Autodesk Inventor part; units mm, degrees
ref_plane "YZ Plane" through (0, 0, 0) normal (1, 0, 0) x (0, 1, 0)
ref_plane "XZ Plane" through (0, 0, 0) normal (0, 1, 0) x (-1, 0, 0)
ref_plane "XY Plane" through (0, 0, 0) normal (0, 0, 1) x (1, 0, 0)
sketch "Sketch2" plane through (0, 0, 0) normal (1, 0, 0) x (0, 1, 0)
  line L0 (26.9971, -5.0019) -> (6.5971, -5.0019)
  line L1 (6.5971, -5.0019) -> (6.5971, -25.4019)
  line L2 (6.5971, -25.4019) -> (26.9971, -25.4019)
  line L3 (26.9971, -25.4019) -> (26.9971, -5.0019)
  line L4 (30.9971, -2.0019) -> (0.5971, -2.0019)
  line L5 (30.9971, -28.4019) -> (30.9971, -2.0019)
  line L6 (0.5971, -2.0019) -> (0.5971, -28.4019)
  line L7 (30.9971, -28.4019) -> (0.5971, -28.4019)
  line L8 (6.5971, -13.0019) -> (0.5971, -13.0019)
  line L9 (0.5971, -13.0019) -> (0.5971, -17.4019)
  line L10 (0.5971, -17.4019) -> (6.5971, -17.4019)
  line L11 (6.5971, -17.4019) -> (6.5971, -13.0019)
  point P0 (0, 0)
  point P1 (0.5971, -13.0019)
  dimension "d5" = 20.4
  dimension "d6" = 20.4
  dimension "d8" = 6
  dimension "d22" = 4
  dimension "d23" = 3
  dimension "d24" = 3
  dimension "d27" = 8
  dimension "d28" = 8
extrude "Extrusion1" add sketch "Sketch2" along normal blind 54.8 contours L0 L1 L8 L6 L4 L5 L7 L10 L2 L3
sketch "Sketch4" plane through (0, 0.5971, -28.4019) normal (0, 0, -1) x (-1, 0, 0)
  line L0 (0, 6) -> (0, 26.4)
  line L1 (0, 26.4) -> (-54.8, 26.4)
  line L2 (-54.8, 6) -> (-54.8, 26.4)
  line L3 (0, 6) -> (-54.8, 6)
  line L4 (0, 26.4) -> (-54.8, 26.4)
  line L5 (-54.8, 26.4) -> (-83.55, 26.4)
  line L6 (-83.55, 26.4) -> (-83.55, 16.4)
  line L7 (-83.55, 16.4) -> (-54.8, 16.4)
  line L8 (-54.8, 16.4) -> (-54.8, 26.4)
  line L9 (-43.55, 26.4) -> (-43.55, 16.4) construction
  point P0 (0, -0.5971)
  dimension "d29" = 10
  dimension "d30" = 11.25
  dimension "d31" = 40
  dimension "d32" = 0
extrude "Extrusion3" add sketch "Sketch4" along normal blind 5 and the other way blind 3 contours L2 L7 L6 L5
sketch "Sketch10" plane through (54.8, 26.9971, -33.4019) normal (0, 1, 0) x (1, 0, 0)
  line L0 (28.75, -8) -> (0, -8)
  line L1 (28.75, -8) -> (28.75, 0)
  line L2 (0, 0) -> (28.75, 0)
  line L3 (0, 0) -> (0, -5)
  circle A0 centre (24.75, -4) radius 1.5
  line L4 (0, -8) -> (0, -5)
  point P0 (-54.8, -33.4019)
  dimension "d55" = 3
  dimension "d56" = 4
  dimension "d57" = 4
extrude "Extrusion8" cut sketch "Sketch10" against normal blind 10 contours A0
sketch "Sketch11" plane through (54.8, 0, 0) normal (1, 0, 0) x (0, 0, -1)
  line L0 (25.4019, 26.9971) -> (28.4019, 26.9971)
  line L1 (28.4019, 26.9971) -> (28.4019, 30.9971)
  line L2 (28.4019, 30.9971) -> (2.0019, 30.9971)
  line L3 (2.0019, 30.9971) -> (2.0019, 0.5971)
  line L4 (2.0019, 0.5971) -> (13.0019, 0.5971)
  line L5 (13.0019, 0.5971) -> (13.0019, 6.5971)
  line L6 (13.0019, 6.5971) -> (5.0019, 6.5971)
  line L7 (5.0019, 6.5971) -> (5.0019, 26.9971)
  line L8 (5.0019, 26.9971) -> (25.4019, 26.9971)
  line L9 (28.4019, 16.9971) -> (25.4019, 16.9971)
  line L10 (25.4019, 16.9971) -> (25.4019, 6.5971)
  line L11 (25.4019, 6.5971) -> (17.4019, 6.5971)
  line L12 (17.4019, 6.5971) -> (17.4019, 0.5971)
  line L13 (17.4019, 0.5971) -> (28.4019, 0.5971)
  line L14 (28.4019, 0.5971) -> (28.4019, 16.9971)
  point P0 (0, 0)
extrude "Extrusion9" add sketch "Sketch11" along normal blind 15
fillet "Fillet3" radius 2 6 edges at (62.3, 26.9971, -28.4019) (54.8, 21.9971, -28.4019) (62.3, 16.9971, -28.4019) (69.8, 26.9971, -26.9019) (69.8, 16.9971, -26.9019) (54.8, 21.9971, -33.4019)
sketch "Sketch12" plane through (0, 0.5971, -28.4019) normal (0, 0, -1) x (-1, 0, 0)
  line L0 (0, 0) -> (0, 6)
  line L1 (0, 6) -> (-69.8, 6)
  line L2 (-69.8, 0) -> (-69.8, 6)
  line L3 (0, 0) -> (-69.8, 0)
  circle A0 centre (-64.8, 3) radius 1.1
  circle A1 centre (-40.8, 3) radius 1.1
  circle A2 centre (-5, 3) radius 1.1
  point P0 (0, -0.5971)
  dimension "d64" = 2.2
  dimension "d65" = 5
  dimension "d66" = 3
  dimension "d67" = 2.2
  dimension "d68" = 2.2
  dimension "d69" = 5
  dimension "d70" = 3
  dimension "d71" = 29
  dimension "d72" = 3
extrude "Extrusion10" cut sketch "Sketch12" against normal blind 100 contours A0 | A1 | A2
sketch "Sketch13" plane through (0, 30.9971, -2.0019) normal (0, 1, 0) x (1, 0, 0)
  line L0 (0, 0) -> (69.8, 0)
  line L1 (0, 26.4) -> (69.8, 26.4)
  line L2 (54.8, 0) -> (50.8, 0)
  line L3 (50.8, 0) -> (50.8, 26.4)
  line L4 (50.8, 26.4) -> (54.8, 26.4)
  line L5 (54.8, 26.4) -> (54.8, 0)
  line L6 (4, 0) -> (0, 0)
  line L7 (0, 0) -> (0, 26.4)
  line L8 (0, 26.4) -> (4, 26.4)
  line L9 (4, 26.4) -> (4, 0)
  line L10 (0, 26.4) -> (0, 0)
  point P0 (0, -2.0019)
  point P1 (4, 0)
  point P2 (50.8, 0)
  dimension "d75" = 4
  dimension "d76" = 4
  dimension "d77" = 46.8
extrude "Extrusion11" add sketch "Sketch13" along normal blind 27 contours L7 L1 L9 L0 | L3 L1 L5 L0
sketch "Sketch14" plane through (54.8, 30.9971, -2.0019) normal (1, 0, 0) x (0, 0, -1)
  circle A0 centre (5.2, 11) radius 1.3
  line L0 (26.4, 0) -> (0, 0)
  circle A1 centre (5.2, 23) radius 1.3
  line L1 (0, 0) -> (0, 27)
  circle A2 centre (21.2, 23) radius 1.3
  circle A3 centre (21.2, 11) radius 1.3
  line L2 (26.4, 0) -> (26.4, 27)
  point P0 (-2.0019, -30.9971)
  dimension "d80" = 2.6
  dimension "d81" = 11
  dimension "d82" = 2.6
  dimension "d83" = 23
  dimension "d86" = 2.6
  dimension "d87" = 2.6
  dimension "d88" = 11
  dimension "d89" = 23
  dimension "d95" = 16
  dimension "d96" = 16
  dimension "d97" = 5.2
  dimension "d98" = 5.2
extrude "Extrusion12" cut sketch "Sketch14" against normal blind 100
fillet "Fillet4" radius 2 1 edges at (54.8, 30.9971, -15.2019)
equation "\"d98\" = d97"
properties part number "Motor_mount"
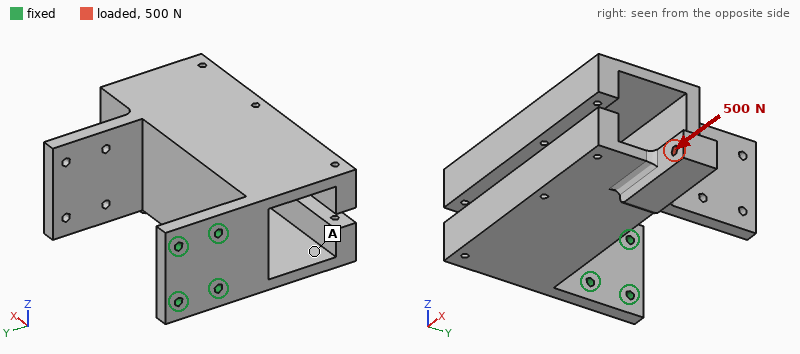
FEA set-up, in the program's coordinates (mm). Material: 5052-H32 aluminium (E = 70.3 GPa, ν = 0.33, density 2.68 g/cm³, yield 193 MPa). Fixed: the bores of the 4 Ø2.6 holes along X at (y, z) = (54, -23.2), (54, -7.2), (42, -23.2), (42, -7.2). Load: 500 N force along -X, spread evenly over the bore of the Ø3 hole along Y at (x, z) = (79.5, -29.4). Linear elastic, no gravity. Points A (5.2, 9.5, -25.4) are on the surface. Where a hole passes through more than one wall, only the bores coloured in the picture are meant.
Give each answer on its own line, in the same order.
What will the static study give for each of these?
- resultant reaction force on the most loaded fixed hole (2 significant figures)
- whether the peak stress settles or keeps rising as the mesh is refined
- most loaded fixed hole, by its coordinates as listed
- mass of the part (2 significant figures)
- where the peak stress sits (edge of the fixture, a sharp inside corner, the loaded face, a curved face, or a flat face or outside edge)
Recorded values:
780 N
keeps rising
(42, -23.2)
86 g
edge of the fixture
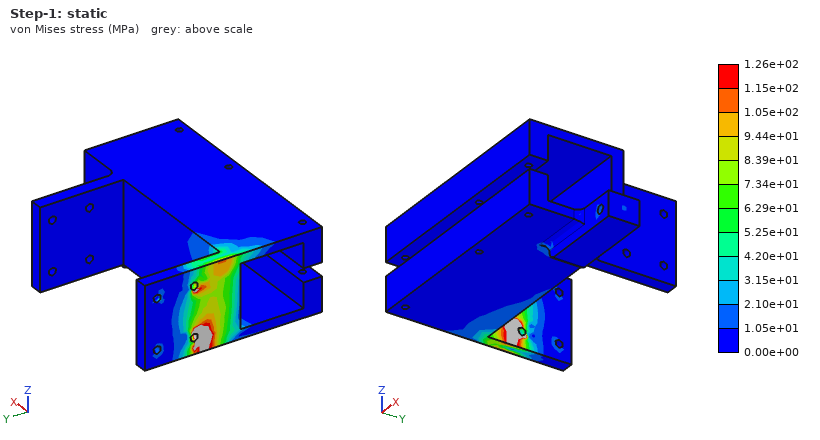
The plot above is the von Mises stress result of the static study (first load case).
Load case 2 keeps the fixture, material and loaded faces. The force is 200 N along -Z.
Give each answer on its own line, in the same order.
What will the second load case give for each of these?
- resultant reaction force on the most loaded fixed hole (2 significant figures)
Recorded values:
910 N
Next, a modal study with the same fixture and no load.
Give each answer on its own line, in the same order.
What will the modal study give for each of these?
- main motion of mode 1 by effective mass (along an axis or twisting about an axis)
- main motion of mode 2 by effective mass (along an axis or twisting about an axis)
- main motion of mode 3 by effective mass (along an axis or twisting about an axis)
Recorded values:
along Y
along Z
twisting about X
